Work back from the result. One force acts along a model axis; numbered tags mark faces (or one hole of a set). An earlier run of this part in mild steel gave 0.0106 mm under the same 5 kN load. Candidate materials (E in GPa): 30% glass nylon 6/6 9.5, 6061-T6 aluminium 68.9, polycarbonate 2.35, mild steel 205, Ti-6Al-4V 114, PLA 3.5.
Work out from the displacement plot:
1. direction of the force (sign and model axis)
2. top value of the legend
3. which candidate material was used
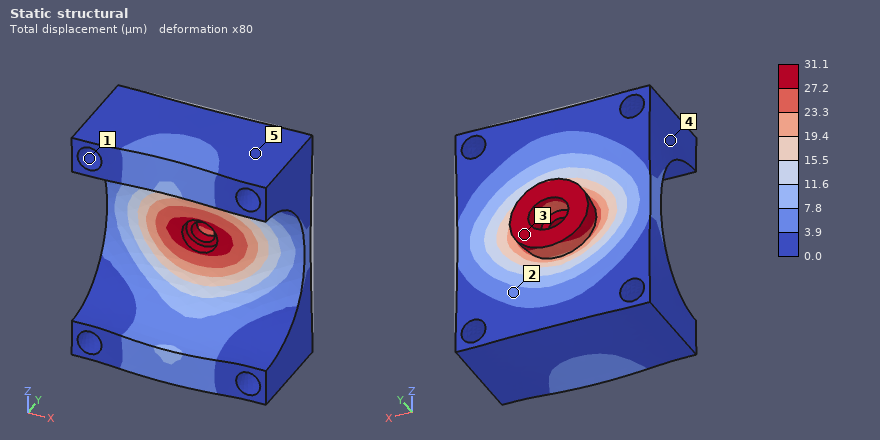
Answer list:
-Y
31.1 µm
6061-T6 aluminium
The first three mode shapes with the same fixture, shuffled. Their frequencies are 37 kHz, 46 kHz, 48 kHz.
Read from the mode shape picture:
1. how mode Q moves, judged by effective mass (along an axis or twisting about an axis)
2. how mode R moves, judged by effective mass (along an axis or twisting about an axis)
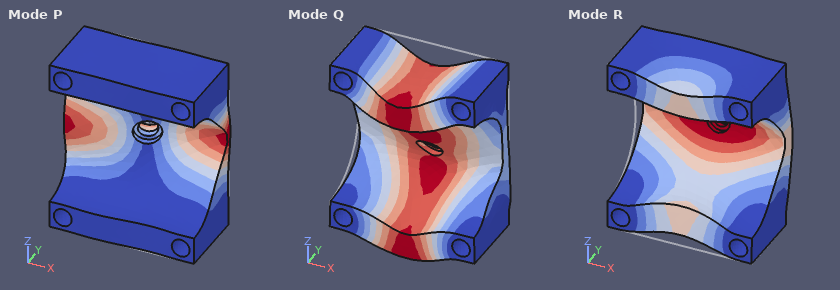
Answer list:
along Z
along Y
